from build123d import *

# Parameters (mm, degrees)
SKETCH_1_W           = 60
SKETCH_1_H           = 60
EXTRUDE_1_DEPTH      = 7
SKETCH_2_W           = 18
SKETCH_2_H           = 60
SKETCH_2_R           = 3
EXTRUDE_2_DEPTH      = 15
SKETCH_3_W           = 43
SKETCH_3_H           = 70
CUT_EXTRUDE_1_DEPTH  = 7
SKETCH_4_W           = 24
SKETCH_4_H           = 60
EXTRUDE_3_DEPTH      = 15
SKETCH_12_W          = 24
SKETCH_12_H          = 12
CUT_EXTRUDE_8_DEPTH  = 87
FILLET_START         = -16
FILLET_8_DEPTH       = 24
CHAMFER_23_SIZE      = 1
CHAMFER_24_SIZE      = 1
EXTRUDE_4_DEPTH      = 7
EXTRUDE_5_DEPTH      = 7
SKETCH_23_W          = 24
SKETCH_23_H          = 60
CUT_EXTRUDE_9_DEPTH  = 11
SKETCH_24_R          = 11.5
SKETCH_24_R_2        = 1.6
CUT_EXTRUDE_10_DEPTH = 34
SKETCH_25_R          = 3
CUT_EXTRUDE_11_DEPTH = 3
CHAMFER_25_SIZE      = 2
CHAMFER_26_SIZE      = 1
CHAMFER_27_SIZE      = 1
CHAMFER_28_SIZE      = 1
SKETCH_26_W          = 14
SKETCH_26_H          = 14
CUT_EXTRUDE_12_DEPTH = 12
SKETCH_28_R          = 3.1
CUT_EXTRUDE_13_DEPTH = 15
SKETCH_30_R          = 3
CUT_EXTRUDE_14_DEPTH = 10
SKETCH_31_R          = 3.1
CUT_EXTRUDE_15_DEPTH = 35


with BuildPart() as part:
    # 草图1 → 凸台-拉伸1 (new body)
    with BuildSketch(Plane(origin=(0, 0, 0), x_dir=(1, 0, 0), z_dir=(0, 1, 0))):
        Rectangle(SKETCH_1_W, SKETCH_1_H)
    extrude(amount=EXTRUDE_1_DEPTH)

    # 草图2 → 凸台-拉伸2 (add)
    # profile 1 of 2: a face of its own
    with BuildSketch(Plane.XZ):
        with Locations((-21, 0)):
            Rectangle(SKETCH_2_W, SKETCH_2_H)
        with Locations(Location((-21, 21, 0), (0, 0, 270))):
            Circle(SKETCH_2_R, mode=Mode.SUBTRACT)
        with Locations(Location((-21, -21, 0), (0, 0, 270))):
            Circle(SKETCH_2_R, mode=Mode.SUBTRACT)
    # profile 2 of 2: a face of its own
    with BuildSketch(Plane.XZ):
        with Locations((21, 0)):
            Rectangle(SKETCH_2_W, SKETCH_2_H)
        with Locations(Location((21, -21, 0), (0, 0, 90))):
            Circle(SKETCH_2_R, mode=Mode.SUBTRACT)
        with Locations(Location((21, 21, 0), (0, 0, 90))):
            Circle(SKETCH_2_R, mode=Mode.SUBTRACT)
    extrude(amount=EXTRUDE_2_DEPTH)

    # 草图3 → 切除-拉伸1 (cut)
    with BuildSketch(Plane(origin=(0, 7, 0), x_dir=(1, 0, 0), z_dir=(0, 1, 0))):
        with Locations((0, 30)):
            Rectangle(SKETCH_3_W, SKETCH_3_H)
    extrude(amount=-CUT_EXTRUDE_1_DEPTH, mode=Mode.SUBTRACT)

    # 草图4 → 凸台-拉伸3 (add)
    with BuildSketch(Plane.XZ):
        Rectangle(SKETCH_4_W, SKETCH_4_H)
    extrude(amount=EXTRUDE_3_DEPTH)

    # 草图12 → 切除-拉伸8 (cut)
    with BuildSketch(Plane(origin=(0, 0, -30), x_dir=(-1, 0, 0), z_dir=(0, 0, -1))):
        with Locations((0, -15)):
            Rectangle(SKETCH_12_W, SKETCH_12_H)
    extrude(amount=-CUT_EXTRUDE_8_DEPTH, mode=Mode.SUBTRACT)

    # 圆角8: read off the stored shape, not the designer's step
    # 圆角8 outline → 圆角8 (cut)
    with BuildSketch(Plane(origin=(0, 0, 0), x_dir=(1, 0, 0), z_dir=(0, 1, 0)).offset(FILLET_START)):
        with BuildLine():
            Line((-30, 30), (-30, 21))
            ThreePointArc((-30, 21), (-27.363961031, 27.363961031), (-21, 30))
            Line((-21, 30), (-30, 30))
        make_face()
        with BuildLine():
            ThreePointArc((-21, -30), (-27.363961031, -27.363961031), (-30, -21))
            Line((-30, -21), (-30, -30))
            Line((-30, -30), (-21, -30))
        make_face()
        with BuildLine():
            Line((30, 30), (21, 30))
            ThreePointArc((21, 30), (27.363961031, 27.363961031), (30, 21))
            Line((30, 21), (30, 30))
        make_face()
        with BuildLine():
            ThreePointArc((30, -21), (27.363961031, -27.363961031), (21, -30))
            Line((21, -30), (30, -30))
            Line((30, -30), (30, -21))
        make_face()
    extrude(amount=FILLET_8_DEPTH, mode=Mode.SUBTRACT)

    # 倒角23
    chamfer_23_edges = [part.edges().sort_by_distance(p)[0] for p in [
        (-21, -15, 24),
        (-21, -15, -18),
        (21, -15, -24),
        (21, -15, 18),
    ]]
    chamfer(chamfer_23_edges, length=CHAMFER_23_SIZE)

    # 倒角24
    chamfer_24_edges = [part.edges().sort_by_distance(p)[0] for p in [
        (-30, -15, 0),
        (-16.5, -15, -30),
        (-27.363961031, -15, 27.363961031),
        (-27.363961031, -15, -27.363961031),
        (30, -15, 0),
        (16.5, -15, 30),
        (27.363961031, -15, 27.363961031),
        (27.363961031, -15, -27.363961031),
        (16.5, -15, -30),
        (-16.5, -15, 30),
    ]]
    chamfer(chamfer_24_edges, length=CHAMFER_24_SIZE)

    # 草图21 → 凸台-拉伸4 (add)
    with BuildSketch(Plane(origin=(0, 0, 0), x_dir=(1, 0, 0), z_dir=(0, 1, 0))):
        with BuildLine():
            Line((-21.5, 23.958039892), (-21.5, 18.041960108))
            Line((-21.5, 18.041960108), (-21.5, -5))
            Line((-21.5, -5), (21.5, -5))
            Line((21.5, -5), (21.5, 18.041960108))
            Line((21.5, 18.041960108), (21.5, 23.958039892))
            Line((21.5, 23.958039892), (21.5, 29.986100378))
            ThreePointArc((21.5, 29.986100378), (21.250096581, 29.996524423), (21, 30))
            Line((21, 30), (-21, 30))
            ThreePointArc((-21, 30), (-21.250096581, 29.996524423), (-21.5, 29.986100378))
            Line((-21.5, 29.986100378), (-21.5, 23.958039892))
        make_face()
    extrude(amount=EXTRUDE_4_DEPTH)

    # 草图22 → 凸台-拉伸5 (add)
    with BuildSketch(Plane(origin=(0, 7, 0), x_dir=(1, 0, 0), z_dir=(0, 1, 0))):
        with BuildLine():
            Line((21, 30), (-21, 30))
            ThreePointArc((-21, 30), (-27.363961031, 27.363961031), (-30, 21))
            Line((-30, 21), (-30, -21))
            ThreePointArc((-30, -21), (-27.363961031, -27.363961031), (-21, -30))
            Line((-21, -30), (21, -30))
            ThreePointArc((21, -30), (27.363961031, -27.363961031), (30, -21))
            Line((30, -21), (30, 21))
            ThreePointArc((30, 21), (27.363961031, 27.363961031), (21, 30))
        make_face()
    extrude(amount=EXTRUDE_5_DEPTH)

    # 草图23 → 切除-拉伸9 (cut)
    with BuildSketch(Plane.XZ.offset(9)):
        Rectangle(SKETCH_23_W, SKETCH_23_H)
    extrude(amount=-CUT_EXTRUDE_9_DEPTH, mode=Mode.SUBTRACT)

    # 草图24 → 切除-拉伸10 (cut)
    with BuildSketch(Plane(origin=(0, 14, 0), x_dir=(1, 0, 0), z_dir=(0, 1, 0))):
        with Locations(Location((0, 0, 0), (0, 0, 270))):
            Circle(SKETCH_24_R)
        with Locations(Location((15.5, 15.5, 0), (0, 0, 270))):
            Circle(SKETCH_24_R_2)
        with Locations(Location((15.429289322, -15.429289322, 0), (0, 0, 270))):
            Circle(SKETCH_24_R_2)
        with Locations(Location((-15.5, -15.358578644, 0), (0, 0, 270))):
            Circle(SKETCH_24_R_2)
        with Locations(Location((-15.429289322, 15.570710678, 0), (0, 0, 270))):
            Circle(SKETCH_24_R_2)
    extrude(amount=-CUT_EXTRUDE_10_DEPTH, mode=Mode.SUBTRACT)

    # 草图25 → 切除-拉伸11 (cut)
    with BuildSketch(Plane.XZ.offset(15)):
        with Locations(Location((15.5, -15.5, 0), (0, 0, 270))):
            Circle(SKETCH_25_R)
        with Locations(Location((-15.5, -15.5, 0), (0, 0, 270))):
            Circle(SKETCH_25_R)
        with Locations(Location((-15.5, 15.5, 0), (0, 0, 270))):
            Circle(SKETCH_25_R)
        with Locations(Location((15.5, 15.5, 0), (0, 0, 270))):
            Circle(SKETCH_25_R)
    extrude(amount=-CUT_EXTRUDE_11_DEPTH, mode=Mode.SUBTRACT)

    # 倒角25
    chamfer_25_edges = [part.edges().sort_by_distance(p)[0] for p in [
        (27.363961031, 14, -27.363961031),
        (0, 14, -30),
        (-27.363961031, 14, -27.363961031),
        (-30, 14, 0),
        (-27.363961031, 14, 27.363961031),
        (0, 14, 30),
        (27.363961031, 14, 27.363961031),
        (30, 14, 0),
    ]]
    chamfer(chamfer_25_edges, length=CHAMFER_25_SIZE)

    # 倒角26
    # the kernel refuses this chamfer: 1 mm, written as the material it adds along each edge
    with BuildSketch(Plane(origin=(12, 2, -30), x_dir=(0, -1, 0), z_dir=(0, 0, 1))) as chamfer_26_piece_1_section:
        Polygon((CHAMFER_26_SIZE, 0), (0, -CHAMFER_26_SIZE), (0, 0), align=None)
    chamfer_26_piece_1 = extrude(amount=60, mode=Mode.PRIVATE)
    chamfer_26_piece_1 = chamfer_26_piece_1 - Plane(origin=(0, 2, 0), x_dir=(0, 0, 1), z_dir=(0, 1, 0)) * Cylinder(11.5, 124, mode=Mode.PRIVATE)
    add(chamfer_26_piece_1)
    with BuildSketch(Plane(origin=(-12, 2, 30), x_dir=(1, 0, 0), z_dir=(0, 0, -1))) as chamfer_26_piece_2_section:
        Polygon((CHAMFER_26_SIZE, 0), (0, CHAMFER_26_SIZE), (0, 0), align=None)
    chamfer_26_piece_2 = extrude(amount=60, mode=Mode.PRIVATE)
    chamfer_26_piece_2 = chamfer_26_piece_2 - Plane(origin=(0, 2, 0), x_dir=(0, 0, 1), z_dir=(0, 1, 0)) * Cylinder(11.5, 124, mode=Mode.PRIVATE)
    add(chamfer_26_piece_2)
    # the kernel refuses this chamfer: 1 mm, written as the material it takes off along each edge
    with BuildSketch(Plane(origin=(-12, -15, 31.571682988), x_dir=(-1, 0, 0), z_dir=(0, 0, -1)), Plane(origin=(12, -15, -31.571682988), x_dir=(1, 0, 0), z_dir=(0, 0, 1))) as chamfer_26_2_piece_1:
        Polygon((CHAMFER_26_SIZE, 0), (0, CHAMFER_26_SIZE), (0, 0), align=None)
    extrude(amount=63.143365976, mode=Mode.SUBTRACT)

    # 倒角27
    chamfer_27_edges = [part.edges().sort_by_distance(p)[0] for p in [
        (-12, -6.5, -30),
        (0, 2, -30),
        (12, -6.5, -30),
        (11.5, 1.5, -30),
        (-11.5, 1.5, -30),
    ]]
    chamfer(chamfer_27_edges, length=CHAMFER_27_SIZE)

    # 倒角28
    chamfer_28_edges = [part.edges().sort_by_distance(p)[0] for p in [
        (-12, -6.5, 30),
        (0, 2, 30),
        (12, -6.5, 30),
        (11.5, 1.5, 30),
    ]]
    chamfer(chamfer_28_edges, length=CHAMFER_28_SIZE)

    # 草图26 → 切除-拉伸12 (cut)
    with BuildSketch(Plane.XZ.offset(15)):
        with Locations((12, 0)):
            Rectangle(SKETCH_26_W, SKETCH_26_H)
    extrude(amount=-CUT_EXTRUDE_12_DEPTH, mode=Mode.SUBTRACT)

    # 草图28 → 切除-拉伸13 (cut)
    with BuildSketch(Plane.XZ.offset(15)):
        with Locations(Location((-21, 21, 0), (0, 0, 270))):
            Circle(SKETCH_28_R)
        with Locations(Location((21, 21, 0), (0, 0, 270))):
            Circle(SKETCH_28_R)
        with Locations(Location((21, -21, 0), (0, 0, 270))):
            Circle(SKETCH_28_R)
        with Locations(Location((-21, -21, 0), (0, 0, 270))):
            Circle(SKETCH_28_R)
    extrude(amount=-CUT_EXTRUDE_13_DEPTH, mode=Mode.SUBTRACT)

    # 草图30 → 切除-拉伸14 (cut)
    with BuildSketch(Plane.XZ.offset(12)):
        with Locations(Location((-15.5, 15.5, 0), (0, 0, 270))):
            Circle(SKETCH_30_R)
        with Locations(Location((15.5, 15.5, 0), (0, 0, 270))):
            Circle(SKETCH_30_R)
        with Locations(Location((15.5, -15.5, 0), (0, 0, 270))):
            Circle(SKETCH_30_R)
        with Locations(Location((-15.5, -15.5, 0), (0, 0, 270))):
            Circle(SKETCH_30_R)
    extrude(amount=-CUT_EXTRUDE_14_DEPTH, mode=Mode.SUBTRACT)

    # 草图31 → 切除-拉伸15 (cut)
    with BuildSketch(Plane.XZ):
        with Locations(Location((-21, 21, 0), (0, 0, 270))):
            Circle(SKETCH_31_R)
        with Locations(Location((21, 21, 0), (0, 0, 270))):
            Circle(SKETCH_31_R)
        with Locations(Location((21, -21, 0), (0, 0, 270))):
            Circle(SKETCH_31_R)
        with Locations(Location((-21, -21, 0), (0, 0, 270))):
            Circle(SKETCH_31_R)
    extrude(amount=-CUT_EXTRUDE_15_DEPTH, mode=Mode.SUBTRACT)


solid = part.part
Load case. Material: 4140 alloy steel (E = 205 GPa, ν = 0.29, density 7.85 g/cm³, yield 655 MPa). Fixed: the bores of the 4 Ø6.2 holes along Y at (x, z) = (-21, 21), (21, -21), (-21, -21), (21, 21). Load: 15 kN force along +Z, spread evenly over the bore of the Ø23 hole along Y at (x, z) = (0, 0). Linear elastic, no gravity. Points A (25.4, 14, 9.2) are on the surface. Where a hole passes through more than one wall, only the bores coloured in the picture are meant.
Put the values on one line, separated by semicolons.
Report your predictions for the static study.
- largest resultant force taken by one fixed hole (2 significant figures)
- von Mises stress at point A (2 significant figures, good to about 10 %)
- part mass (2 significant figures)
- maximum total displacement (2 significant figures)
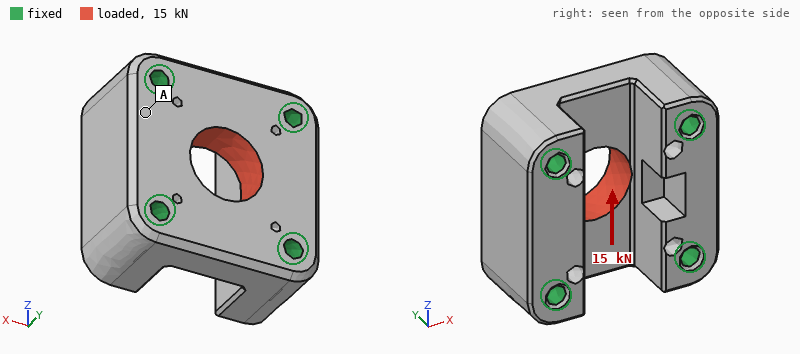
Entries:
4.1 kN; 4.5 MPa; 520 g; 2.8 µm
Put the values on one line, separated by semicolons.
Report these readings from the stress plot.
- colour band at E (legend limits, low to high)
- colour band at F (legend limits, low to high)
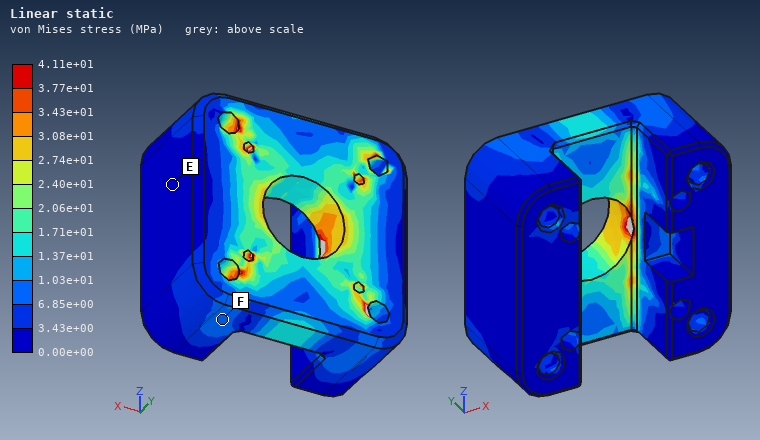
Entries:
0.00e+00 to 3.43e+00 MPa; 6.85e+00 to 1.03e+01 MPa
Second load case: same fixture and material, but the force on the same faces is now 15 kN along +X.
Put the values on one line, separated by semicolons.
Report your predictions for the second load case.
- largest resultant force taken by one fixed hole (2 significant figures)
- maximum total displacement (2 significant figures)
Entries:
4.0 kN; 3.1 µm
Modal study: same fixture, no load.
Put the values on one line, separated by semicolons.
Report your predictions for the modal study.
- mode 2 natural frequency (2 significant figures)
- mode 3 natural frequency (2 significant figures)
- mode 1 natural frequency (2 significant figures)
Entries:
29 kHz; 30 kHz; 27 kHz
